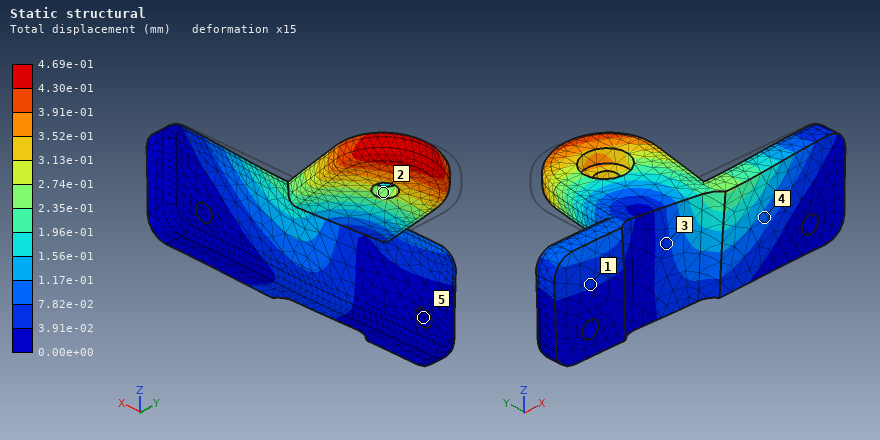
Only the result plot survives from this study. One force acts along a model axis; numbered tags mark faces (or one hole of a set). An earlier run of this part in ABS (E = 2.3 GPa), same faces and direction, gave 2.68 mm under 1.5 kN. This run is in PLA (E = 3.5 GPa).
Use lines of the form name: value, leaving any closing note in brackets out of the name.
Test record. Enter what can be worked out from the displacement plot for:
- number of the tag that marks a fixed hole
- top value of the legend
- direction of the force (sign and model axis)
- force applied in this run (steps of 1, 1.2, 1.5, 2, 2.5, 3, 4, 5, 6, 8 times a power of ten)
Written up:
number of the tag that marks a fixed hole: 5
top value of the legend: 4.69e-01 mm
direction of the force: +X
force applied in this run: 400 N
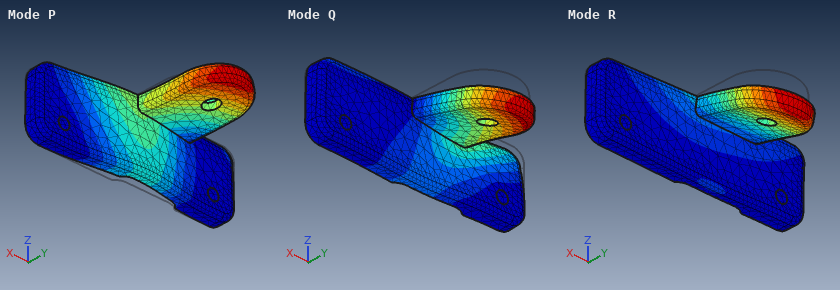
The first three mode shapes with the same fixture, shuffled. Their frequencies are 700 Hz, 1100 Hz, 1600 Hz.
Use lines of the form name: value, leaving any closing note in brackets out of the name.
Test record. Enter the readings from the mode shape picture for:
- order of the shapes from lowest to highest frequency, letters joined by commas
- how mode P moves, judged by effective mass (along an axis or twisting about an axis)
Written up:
order of the shapes from lowest to highest frequency, letters joined by commas: R, P, Q
how mode P moves, judged by effective mass: along Y
